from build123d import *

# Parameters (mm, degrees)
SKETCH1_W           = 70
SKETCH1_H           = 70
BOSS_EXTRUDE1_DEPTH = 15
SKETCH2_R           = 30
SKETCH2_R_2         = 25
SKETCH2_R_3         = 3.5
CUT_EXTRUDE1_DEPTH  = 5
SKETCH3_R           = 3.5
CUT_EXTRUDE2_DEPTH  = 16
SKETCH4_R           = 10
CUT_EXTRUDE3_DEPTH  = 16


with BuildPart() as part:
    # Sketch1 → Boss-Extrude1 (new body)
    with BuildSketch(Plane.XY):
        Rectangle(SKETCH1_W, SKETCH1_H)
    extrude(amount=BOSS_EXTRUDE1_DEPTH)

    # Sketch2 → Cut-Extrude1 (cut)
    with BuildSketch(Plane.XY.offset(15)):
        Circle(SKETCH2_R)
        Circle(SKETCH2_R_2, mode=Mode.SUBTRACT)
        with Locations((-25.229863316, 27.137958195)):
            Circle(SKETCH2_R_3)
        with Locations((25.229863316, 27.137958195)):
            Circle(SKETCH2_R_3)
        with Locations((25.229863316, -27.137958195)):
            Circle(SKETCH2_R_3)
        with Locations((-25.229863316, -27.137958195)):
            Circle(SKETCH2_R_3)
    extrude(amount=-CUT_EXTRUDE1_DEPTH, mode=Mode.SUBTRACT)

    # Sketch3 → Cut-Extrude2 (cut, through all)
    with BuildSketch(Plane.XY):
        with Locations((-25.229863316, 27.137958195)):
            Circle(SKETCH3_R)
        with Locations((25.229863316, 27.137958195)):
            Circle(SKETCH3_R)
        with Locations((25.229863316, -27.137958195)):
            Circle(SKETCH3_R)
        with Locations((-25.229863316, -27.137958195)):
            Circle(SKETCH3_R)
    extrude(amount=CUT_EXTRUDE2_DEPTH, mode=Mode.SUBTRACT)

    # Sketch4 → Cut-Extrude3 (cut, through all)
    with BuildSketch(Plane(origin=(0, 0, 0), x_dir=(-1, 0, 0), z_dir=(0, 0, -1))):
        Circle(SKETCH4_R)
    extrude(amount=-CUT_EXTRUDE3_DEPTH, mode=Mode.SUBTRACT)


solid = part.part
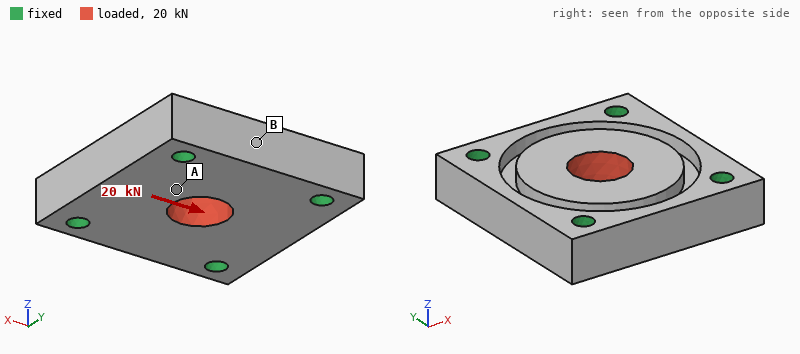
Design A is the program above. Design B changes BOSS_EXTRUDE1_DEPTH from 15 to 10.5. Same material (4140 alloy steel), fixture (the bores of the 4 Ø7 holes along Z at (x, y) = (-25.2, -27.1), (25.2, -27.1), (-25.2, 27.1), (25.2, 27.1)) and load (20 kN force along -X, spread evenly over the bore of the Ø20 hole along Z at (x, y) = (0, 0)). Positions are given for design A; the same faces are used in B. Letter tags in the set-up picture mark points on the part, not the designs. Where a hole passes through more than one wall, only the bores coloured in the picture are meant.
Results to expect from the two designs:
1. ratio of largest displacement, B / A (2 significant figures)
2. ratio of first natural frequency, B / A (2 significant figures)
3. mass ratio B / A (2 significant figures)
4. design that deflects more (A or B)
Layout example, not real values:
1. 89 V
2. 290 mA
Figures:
1. 1.1
2. 0.87
3. 0.74
4. B
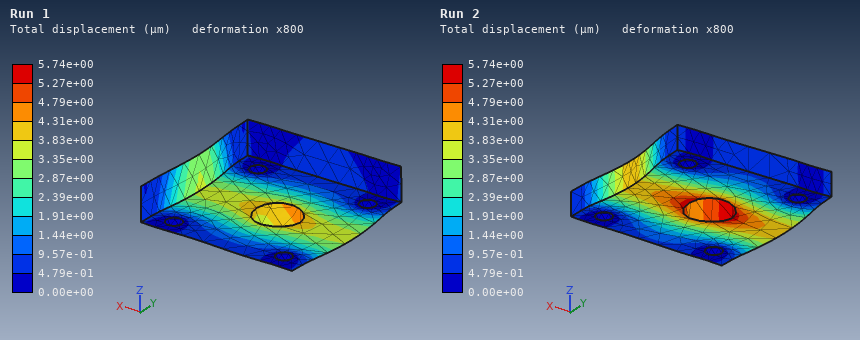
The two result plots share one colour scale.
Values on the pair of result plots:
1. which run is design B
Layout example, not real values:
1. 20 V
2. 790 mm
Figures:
1. Run 2
